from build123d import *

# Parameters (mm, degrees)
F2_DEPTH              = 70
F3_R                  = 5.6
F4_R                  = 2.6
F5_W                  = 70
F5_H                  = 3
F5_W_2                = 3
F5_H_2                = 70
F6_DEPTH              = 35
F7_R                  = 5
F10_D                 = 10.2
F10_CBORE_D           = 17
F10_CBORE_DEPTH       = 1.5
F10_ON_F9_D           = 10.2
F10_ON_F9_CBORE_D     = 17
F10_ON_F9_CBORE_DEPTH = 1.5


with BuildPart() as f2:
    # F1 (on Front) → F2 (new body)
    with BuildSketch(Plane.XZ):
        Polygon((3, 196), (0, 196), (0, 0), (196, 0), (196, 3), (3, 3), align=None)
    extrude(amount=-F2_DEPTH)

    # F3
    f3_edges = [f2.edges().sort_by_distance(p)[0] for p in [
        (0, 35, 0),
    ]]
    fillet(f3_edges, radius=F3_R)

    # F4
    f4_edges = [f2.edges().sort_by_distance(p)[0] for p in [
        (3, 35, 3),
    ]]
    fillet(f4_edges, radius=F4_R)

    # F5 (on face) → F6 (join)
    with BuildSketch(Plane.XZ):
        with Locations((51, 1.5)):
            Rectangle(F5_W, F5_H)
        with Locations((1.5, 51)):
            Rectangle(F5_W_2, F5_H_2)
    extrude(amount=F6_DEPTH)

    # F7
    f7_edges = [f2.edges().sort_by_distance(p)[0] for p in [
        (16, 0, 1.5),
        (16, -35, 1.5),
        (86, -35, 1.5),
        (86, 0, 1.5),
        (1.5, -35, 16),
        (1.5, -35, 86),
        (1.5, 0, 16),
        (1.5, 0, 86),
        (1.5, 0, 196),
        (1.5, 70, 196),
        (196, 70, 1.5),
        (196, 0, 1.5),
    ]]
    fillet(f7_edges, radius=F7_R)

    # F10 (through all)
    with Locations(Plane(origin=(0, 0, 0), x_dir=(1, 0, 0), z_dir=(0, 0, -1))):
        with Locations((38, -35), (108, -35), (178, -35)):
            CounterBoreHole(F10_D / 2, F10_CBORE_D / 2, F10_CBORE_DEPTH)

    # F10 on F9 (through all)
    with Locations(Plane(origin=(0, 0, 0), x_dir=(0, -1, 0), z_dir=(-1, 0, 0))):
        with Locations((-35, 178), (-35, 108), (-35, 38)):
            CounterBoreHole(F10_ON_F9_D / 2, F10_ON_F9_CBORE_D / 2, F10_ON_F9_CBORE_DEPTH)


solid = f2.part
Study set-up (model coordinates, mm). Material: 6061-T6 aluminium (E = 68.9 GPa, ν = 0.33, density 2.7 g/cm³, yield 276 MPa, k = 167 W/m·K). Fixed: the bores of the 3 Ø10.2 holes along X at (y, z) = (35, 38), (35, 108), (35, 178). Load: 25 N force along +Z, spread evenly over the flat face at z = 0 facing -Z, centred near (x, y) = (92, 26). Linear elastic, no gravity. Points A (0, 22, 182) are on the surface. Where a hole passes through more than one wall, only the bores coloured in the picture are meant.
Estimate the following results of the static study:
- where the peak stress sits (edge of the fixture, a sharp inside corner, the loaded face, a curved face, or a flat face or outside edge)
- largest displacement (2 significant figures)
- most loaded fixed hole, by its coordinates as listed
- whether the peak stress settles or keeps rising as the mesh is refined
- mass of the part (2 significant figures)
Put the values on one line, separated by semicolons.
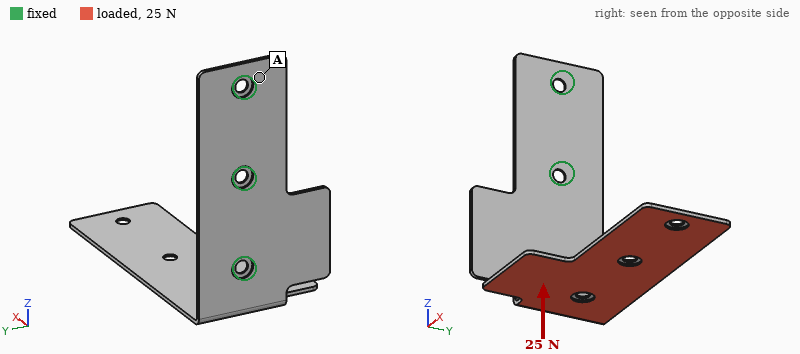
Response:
edge of the fixture; 3.1 mm; (35, 38); keeps rising; 250 g
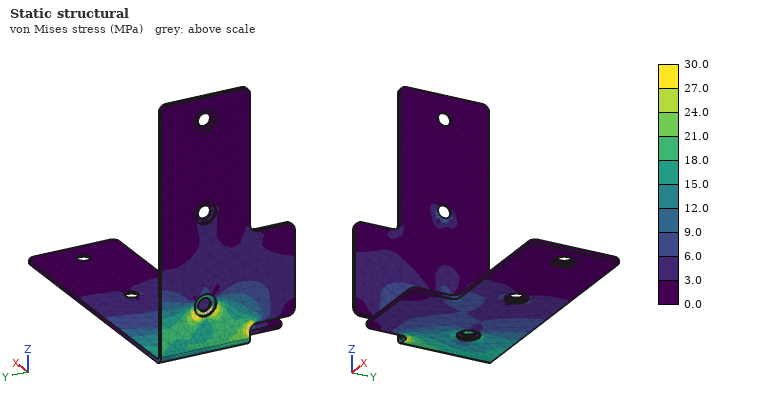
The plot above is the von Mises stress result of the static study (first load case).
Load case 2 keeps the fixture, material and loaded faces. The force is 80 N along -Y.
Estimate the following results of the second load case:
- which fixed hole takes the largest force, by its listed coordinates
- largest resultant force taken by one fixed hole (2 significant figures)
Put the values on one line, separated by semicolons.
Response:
(35, 38); 180 N
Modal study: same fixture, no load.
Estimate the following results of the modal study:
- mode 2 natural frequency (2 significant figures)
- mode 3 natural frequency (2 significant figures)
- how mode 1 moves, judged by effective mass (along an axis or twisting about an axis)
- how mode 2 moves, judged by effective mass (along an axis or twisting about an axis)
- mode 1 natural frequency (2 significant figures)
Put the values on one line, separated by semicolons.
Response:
86 Hz; 270 Hz; along Z; along Y; 51 Hz
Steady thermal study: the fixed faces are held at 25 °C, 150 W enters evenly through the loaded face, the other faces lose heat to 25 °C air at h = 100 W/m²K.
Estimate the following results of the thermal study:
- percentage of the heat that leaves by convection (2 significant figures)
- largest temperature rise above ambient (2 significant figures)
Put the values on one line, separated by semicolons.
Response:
90 %; 76 K
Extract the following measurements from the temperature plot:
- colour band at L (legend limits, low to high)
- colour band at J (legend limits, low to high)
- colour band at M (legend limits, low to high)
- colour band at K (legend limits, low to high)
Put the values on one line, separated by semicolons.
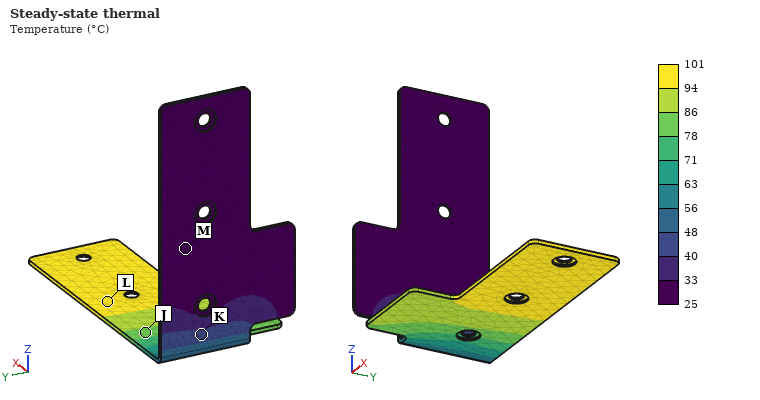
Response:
94 to 101 °C; 78 to 86 °C; 25 to 33 °C; 40 to 48 °C
